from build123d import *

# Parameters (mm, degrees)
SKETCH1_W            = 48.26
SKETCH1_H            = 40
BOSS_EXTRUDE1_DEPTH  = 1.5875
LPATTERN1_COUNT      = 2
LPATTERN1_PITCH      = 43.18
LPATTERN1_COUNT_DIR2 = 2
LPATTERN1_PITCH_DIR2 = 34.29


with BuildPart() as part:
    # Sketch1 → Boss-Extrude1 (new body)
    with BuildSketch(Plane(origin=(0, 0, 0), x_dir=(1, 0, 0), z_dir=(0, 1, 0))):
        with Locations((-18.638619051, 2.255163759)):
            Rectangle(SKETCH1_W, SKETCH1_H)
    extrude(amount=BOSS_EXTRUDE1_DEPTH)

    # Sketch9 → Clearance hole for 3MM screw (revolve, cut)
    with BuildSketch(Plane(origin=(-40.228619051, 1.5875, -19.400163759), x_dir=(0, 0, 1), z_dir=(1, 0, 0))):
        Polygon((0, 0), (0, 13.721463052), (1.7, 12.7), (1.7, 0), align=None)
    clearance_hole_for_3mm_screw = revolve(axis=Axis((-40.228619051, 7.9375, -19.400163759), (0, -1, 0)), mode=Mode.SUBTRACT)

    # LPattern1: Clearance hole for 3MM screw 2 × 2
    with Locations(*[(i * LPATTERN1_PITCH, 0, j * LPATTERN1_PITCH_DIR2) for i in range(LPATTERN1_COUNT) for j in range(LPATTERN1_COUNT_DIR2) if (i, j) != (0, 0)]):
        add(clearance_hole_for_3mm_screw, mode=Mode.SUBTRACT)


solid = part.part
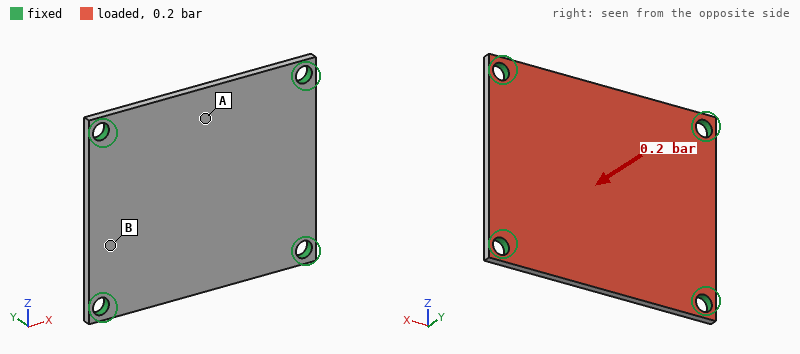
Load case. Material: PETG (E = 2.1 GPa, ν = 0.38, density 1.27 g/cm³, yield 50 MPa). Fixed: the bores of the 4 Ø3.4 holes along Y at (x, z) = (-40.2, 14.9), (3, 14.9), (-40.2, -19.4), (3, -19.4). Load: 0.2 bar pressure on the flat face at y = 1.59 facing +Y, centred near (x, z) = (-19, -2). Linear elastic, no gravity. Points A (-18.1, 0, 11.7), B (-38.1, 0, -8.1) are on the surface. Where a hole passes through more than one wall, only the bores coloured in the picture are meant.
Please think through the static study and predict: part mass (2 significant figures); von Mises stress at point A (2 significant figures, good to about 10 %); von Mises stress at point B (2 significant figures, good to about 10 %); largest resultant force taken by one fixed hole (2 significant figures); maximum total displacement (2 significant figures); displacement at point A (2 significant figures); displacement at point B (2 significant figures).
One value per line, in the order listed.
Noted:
3.8 g
4.0 MPa
2.1 MPa
9.5 N
0.39 mm
0.32 mm
0.12 mm
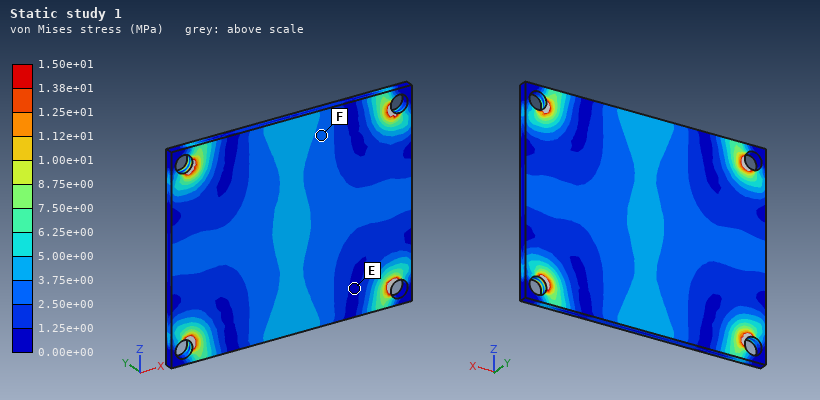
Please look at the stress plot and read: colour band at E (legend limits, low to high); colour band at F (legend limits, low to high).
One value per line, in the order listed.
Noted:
0.00e+00 to 1.25e+00 MPa
2.50e+00 to 3.75e+00 MPa
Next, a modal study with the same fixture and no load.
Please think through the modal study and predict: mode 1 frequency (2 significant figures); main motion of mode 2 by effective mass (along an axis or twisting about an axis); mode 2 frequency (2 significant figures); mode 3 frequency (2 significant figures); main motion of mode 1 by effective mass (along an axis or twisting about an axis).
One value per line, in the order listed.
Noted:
950 Hz
twisting about X
1500 Hz
2000 Hz
along Y
